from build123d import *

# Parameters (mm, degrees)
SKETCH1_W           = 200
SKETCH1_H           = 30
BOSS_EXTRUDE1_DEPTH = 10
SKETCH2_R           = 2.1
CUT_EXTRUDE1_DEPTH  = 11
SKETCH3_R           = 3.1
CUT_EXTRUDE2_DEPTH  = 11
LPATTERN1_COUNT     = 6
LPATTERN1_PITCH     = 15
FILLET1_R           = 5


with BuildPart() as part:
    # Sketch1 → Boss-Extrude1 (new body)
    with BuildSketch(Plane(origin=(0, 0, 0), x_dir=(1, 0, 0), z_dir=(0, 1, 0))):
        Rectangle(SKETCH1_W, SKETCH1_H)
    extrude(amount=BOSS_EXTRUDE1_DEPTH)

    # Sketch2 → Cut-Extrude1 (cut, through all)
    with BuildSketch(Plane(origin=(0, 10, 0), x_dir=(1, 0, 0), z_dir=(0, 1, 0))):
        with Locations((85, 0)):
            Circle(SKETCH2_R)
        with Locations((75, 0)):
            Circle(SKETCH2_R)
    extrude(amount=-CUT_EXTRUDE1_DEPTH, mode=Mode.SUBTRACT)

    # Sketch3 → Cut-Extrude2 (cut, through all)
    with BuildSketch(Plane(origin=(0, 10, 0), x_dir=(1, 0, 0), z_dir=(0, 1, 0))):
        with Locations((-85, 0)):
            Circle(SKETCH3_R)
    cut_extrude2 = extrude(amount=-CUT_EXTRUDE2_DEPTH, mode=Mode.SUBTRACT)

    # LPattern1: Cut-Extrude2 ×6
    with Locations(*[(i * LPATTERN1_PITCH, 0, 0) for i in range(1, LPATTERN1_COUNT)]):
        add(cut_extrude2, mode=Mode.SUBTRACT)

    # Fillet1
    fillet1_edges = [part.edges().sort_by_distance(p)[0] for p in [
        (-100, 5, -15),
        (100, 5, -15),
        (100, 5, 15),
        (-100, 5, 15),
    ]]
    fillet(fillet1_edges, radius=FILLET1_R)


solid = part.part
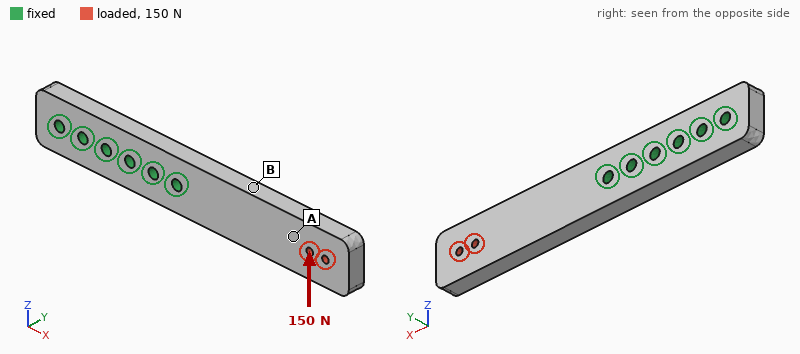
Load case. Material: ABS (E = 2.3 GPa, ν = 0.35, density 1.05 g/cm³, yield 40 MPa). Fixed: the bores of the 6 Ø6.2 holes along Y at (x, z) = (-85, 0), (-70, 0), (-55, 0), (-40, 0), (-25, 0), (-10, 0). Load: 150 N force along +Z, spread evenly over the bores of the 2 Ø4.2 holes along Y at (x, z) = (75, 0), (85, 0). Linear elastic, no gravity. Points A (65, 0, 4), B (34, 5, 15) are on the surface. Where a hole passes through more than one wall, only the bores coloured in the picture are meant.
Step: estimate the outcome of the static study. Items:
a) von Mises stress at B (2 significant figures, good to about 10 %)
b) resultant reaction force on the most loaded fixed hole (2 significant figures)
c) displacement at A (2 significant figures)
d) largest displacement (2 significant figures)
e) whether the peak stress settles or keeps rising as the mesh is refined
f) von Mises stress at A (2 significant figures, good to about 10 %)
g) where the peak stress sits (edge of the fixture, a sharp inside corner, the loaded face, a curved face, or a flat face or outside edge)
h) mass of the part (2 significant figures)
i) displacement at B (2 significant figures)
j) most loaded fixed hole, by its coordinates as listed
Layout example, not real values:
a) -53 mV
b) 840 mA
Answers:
a) 4.6 MPa
b) 550 N
c) 0.81 mm
d) 1.4 mm
e) keeps rising
f) 1.3 MPa
g) edge of the fixture
h) 61 g
i) 0.42 mm
j) (-10, 0)
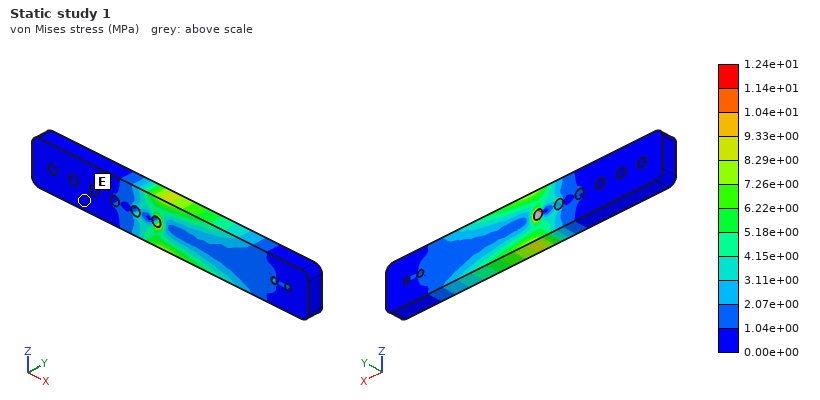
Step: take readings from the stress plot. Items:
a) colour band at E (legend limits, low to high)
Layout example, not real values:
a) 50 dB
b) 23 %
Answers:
a) 0.00e+00 to 1.04e+00 MPa
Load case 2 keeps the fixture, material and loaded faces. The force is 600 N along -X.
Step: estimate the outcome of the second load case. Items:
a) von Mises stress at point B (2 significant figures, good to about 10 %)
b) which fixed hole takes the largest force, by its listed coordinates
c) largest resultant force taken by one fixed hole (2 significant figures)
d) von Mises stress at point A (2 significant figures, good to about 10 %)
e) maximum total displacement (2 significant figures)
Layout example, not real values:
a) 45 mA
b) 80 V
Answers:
a) 2.0 MPa
b) (-10, 0)
c) 450 N
d) 2.4 MPa
e) 91 µm
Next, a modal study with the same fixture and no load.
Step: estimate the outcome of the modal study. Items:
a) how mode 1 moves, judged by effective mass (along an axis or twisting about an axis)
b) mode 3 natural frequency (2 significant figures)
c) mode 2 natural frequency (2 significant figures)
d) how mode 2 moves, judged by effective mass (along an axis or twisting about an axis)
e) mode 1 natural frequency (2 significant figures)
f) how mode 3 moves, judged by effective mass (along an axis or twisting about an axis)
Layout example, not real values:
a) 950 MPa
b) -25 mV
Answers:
a) along Y
b) 1200 Hz
c) 480 Hz
d) along Z
e) 200 Hz
f) twisting about X
